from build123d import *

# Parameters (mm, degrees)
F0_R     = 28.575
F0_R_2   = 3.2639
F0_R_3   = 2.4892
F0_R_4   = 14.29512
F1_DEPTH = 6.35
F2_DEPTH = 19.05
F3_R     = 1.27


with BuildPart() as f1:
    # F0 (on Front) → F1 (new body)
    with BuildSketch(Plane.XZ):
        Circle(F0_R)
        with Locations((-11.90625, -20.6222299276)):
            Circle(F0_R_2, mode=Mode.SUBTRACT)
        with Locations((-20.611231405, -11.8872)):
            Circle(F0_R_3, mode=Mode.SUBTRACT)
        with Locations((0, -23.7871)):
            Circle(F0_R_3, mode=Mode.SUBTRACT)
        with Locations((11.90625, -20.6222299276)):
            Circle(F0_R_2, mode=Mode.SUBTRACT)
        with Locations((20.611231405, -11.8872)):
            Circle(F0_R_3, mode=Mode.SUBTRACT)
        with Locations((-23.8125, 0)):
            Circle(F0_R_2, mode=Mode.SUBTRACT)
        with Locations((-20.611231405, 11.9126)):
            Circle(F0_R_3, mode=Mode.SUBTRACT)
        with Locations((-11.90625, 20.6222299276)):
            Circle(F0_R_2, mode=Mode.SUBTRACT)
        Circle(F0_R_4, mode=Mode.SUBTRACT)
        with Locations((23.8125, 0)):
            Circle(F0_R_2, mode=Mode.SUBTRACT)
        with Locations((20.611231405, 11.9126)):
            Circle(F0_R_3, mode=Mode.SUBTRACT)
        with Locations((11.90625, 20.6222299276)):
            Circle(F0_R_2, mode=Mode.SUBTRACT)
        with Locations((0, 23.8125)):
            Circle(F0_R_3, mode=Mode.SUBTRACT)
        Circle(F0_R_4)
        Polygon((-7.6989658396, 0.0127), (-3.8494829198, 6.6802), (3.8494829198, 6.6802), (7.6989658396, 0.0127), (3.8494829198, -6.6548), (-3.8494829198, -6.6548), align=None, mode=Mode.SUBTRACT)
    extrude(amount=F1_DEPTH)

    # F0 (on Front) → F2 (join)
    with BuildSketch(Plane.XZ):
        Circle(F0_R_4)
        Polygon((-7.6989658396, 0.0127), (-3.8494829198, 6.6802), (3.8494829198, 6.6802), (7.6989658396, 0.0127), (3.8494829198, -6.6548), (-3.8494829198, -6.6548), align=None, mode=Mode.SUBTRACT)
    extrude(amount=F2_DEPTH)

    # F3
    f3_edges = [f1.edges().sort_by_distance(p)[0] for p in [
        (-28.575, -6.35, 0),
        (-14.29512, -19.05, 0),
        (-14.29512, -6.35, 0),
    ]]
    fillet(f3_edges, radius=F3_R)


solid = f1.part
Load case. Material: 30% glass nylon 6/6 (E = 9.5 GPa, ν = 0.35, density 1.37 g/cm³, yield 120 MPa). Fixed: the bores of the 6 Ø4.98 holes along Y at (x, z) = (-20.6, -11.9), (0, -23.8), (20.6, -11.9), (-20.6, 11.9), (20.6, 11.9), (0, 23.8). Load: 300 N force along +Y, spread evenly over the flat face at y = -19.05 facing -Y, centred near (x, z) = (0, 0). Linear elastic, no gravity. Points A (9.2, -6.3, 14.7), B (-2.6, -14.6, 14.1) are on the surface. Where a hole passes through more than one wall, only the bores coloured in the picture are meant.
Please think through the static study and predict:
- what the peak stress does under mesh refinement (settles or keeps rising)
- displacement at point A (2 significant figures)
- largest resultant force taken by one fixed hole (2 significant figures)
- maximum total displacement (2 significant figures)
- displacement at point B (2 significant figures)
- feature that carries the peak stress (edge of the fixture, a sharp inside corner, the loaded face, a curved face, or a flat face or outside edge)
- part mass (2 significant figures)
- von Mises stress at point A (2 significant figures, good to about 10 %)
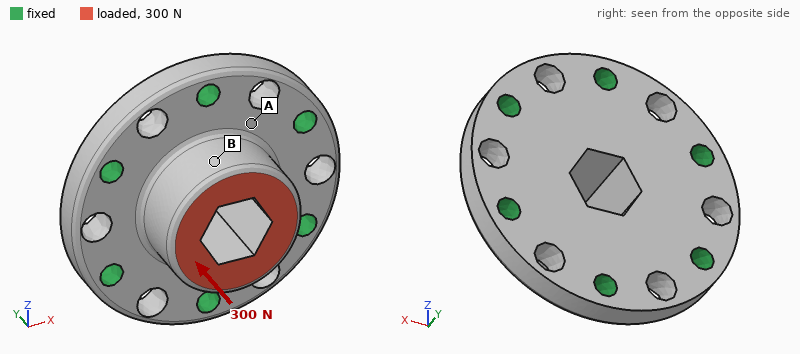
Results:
keeps rising
2.4 µm
56 N
4.7 µm
4.3 µm
edge of the fixture
27 g
0.76 MPa
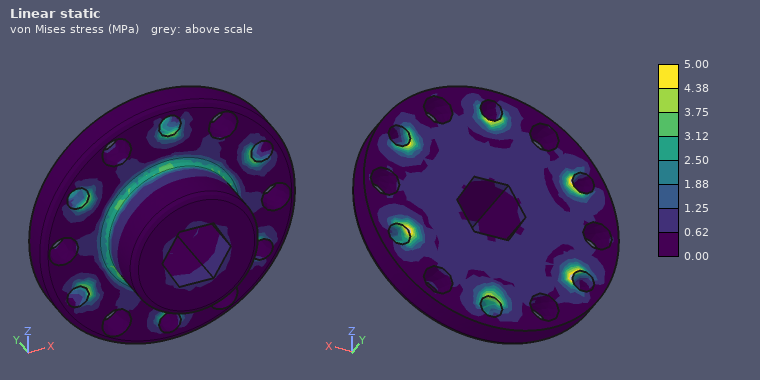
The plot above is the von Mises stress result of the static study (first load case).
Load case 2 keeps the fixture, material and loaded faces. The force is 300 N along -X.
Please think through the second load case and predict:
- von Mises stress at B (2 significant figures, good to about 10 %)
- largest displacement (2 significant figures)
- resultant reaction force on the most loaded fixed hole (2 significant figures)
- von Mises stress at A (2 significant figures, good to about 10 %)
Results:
0.83 MPa
11 µm
98 N
1.5 MPa
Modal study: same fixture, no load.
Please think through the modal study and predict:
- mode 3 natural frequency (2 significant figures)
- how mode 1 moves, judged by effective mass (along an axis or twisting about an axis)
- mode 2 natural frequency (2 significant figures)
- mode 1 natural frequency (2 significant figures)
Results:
13 kHz
along Y
13 kHz
11 kHz
